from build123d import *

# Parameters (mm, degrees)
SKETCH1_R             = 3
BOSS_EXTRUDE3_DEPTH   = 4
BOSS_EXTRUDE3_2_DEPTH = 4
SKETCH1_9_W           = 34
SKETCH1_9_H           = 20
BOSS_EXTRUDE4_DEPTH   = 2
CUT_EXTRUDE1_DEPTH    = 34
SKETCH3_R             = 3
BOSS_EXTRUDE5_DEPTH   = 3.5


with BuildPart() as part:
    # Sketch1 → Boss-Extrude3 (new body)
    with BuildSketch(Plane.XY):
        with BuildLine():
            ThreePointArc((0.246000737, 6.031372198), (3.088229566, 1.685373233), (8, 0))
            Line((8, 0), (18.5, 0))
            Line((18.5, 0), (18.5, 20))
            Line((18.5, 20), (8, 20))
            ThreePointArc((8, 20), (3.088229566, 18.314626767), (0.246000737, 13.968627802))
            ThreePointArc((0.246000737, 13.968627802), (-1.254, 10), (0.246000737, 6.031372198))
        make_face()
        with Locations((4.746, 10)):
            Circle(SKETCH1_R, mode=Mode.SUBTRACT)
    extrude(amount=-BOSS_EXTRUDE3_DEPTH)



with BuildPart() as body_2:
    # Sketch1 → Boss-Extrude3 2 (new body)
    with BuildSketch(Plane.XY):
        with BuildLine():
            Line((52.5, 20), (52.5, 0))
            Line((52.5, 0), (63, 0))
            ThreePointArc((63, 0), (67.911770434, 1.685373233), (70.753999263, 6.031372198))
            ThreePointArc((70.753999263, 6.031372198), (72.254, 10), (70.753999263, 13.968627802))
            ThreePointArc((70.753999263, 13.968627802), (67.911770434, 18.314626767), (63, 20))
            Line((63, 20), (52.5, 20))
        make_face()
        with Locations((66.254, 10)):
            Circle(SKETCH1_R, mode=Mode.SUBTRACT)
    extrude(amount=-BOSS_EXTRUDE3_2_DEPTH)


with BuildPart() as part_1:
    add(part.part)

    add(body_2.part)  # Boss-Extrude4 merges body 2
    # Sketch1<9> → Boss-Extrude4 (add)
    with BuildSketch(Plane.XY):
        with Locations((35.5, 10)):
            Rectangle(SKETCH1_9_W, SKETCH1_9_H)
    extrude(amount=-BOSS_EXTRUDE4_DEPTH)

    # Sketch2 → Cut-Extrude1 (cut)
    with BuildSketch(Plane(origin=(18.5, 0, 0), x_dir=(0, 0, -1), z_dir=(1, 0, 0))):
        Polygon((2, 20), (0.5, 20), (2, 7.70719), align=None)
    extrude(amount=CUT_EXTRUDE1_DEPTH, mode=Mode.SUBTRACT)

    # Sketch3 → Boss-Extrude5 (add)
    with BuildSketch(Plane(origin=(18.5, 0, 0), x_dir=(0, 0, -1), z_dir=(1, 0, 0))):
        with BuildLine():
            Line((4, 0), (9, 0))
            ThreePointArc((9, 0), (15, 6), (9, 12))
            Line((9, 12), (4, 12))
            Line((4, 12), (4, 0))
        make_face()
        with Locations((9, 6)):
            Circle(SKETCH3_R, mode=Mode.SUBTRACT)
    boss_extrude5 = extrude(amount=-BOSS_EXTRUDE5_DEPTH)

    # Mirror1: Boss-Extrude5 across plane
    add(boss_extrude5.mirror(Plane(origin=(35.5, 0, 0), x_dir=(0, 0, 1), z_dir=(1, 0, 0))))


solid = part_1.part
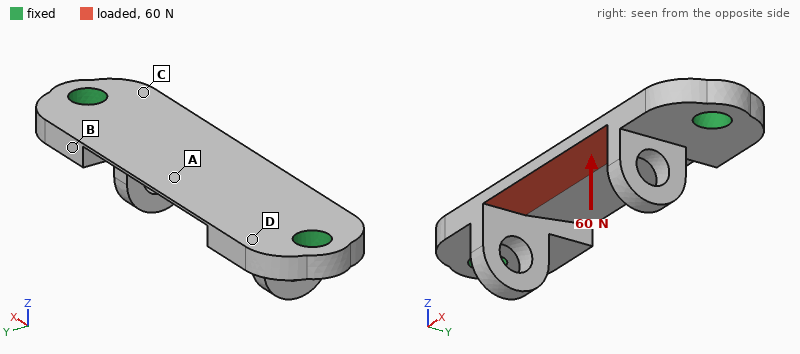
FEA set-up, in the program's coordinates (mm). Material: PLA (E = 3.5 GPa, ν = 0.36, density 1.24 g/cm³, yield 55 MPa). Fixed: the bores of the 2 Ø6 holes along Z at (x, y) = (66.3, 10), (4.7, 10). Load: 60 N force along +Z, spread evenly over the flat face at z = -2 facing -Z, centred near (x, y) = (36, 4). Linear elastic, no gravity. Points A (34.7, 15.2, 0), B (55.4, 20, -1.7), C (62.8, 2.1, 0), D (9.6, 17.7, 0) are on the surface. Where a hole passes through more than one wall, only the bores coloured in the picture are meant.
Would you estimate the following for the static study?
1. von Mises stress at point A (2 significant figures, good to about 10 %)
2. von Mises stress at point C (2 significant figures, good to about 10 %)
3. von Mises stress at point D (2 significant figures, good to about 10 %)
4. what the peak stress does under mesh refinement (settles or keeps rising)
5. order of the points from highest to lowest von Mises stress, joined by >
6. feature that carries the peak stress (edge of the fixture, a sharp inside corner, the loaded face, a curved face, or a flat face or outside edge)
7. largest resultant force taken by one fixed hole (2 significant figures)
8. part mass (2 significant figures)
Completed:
7.7 MPa
5.8 MPa
3.6 MPa
keeps rising
A > C > D > B
edge of the fixture
56 N
5.2 g
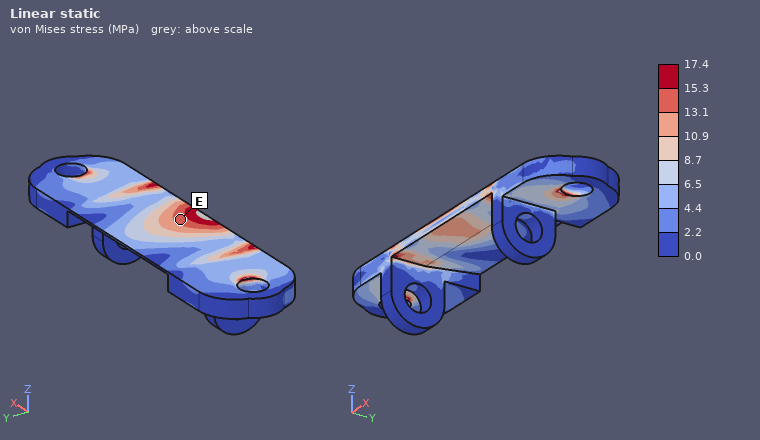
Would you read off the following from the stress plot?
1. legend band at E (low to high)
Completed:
13.1 to 15.3 MPa
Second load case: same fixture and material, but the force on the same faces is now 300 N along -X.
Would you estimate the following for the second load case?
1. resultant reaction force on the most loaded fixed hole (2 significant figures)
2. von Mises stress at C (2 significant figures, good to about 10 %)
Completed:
150 N
4.4 MPa
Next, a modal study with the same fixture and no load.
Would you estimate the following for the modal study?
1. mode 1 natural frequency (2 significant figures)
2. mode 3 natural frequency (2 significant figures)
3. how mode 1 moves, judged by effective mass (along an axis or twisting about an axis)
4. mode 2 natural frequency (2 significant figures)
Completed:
1800 Hz
3200 Hz
along Z
2900 Hz
